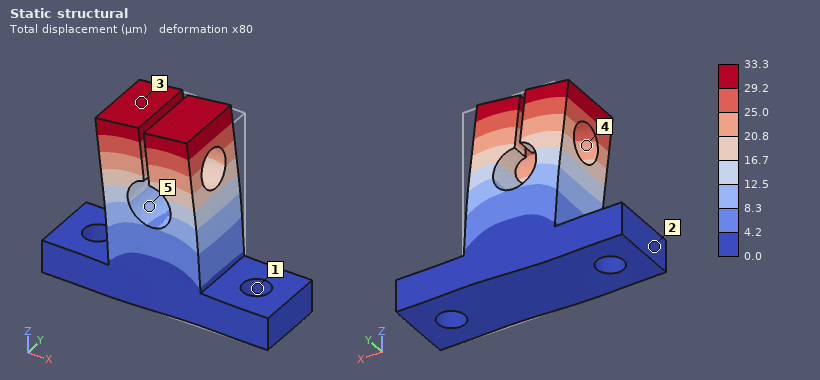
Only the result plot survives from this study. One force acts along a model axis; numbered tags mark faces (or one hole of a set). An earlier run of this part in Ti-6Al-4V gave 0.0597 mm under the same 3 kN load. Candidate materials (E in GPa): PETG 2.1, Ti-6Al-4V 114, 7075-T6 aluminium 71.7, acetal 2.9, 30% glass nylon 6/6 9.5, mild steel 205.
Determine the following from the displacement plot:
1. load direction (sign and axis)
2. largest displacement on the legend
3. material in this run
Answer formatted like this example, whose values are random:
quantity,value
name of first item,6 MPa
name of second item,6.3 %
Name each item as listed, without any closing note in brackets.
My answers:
quantity,value
load direction,-X
largest displacement on the legend,33.3 µm
material in this run,mild steel
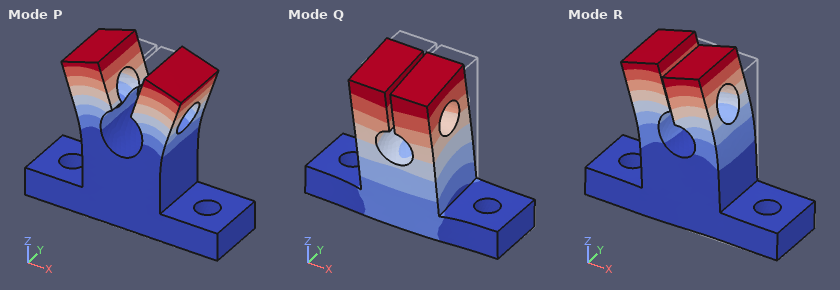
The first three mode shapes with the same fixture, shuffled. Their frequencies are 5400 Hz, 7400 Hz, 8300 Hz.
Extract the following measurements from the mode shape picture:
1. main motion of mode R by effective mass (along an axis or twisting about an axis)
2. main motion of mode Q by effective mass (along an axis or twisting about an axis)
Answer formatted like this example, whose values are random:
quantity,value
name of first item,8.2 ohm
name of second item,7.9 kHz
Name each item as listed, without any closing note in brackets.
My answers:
quantity,value
main motion of mode R by effective mass,along X
main motion of mode Q by effective mass,along Y
